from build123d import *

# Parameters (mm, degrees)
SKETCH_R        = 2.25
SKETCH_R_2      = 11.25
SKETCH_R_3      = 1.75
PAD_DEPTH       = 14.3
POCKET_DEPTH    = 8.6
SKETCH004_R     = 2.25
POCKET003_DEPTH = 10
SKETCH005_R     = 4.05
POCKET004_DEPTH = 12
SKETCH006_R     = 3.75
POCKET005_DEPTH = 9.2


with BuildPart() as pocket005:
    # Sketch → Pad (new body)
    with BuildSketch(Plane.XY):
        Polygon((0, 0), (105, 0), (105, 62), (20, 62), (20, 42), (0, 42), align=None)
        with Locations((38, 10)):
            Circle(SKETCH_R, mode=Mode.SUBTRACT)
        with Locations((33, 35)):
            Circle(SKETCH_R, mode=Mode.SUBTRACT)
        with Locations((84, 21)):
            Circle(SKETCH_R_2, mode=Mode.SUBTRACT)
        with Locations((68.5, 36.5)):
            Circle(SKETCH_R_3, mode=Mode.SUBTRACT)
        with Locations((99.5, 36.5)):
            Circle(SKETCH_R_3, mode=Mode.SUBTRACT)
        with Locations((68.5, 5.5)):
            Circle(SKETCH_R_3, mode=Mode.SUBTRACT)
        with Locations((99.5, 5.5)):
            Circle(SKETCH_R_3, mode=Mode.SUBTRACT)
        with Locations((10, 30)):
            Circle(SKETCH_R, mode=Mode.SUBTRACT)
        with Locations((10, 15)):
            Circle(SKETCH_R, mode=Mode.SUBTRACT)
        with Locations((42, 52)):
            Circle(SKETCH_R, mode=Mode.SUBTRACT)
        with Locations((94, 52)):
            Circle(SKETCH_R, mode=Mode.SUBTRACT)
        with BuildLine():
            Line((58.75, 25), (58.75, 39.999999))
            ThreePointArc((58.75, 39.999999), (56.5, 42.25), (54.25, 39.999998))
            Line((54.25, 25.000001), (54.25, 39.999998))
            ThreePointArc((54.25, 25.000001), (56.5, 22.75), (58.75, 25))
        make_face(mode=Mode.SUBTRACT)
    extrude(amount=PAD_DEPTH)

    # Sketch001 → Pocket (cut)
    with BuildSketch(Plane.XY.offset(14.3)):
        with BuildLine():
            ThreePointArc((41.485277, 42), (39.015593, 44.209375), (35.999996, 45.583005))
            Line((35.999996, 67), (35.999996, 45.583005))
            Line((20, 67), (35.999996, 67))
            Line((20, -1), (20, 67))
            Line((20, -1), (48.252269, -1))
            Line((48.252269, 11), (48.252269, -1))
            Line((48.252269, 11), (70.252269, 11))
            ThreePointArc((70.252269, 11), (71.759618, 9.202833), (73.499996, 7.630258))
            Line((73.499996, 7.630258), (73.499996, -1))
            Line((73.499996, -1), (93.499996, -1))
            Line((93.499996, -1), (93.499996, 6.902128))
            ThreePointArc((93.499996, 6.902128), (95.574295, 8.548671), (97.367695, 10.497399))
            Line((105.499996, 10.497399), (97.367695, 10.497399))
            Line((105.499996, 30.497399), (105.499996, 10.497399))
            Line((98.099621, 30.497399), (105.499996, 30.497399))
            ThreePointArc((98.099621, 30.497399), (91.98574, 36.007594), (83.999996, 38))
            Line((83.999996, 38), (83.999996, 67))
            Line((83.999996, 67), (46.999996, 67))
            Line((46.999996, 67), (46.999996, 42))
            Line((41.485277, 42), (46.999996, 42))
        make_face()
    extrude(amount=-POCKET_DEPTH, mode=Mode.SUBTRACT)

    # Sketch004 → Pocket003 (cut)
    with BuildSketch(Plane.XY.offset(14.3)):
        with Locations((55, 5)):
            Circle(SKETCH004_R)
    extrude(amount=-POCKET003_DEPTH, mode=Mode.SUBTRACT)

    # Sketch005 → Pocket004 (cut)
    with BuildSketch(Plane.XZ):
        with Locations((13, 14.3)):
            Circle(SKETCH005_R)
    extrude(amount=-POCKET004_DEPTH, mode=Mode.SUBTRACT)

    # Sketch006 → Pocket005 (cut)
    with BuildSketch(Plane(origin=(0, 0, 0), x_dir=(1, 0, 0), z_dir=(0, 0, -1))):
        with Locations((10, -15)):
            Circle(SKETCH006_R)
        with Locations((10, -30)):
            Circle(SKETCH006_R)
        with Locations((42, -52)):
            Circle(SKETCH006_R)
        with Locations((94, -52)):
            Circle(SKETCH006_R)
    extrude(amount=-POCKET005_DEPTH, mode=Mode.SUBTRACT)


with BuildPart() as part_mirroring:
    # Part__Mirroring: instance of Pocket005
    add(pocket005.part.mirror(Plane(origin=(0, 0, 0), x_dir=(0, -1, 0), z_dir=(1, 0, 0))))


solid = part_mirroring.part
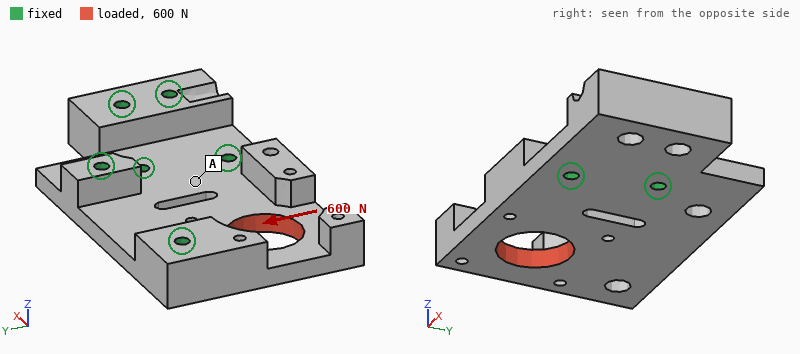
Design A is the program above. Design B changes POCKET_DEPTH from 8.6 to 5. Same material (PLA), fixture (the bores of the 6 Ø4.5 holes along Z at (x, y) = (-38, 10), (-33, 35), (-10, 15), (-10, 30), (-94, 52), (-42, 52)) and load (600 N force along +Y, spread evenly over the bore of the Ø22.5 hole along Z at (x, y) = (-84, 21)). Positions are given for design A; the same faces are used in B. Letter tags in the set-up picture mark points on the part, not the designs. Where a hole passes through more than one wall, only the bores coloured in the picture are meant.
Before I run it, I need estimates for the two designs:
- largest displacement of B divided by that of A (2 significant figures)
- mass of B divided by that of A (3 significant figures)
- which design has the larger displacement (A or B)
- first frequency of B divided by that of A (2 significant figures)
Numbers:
0.53
1.28
A
1.4
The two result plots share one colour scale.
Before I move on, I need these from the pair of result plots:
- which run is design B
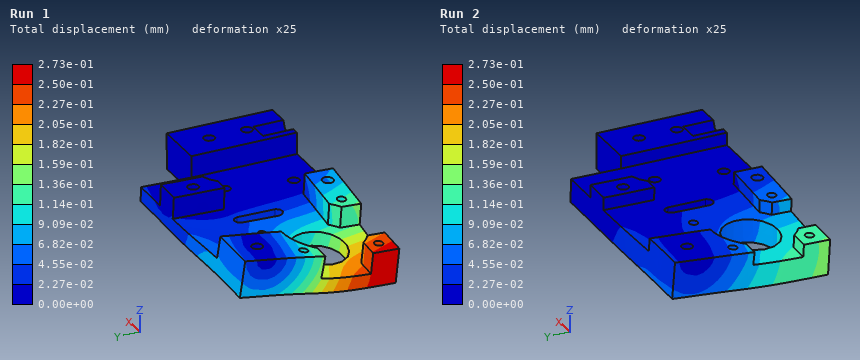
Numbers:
Run 2
